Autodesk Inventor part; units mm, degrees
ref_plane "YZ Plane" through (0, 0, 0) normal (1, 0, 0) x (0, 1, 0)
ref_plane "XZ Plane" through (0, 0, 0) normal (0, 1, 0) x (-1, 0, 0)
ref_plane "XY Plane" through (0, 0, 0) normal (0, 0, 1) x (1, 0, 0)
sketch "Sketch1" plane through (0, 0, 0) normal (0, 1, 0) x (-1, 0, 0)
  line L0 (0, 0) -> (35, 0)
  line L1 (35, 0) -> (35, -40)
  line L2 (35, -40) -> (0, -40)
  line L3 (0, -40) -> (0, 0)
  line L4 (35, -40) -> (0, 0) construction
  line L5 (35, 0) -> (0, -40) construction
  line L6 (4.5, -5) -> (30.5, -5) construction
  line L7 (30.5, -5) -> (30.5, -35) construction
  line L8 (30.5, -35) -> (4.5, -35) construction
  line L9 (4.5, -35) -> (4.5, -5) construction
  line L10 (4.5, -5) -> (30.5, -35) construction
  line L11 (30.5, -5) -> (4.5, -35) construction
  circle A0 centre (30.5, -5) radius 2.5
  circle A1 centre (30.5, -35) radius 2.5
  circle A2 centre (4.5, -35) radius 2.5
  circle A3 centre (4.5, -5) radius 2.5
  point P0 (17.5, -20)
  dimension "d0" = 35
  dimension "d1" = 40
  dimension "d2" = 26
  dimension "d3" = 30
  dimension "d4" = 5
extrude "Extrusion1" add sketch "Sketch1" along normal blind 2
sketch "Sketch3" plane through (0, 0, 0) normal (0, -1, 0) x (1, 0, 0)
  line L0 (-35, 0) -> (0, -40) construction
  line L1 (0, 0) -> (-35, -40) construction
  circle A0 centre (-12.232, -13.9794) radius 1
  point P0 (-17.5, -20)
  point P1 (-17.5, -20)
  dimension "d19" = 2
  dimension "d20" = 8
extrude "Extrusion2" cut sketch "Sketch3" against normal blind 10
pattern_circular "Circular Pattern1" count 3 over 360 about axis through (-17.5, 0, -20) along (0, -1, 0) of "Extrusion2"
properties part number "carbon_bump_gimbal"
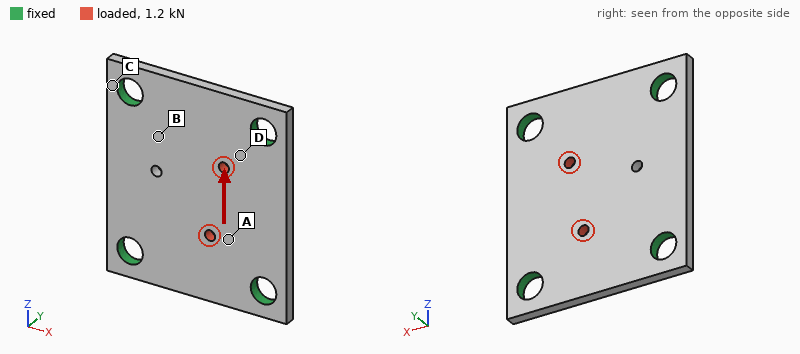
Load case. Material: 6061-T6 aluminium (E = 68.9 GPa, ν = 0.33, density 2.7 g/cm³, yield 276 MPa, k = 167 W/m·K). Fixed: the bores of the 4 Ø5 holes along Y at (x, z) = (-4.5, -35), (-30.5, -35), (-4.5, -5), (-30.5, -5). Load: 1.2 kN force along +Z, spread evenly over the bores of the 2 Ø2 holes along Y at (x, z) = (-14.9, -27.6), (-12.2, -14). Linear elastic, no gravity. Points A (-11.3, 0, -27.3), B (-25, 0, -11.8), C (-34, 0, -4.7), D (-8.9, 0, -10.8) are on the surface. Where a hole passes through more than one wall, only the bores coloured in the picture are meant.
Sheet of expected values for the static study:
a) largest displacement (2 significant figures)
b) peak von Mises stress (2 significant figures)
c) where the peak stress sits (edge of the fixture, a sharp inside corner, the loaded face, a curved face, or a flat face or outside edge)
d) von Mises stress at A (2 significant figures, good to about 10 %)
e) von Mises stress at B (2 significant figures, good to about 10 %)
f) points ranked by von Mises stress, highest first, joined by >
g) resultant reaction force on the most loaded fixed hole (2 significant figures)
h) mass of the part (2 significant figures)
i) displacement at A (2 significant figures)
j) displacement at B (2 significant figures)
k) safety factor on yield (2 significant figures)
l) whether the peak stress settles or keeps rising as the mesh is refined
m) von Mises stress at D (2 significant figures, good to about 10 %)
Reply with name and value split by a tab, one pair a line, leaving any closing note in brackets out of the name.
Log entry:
largest displacement	5.4 µm
peak von Mises stress	85 MPa
where the peak stress sits	the loaded face
von Mises stress at A	17 MPa
von Mises stress at B	10 MPa
points ranked by von Mises stress, highest first, joined by >	D > A > B > C
resultant reaction force on the most loaded fixed hole	420 N
mass of the part	7.1 g
displacement at A	3.1 µm
displacement at B	1.2 µm
safety factor on yield	3.2
whether the peak stress settles or keeps rising as the mesh is refined	settles
von Mises stress at D	26 MPa
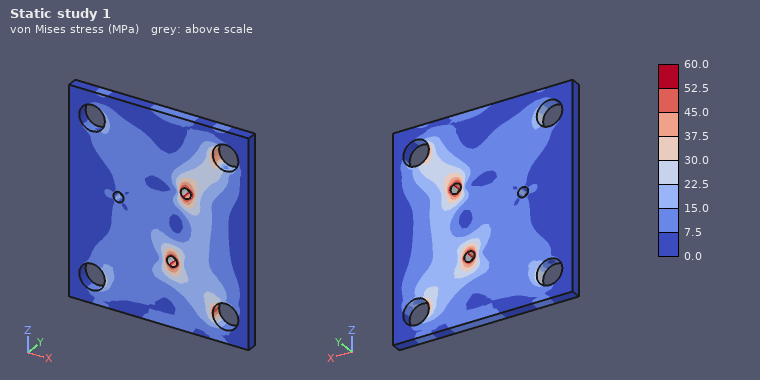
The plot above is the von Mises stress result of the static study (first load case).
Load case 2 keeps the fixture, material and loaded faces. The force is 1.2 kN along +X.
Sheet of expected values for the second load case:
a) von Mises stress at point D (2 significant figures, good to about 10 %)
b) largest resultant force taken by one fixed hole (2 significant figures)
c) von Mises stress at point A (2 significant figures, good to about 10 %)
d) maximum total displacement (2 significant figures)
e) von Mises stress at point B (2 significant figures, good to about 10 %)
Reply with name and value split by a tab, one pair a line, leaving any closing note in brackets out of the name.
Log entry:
von Mises stress at point D	25 MPa
largest resultant force taken by one fixed hole	370 N
von Mises stress at point A	23 MPa
maximum total displacement	5.4 µm
von Mises stress at point B	13 MPa
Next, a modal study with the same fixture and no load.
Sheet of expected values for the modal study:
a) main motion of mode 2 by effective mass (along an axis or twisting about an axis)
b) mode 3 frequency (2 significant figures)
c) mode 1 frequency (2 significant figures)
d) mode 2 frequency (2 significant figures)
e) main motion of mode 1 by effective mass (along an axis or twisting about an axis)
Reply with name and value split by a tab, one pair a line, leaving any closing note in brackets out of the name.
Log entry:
main motion of mode 2 by effective mass	twisting about Z
mode 3 frequency	18 kHz
mode 1 frequency	11 kHz
mode 2 frequency	16 kHz
main motion of mode 1 by effective mass	along Y
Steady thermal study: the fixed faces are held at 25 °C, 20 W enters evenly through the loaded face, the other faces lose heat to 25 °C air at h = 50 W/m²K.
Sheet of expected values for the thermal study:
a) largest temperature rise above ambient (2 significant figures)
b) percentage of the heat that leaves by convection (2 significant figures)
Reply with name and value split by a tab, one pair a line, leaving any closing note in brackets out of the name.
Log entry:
largest temperature rise above ambient	18 K
percentage of the heat that leaves by convection	3.9 %
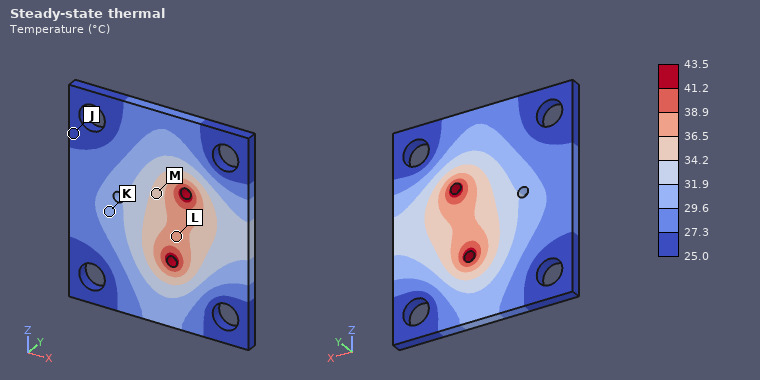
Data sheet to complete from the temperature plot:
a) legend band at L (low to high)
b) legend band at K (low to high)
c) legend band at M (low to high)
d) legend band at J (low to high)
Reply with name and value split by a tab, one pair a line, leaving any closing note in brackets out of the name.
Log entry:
legend band at L	36.5 to 38.9 °C
legend band at K	29.6 to 31.9 °C
legend band at M	34.2 to 36.5 °C
legend band at J	25.0 to 27.3 °C
